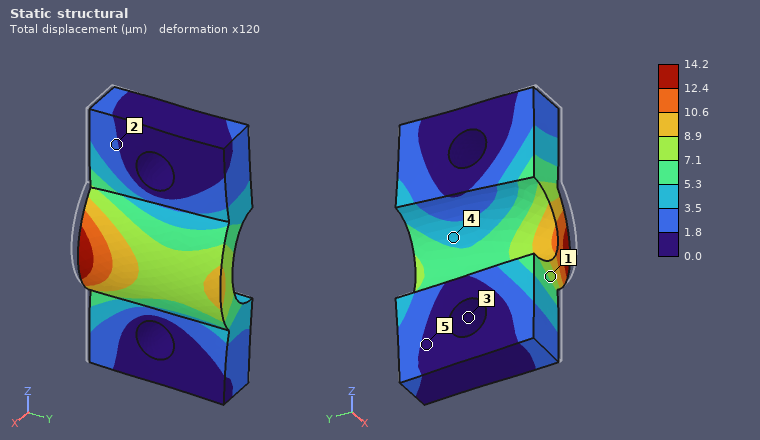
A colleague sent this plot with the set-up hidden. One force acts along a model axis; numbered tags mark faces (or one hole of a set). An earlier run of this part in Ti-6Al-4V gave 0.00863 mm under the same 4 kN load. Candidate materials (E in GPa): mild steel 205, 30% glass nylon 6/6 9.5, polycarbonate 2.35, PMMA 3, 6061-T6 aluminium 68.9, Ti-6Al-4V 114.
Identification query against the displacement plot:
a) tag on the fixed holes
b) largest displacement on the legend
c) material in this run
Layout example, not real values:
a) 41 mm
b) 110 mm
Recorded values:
a) 3
b) 14.2 µm
c) 6061-T6 aluminium
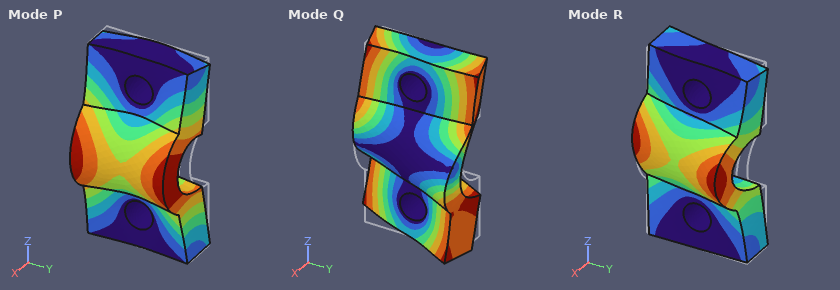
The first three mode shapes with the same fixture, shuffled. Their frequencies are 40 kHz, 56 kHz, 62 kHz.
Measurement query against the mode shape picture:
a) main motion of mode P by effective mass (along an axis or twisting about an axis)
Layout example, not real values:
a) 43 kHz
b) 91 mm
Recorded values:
a) along X
